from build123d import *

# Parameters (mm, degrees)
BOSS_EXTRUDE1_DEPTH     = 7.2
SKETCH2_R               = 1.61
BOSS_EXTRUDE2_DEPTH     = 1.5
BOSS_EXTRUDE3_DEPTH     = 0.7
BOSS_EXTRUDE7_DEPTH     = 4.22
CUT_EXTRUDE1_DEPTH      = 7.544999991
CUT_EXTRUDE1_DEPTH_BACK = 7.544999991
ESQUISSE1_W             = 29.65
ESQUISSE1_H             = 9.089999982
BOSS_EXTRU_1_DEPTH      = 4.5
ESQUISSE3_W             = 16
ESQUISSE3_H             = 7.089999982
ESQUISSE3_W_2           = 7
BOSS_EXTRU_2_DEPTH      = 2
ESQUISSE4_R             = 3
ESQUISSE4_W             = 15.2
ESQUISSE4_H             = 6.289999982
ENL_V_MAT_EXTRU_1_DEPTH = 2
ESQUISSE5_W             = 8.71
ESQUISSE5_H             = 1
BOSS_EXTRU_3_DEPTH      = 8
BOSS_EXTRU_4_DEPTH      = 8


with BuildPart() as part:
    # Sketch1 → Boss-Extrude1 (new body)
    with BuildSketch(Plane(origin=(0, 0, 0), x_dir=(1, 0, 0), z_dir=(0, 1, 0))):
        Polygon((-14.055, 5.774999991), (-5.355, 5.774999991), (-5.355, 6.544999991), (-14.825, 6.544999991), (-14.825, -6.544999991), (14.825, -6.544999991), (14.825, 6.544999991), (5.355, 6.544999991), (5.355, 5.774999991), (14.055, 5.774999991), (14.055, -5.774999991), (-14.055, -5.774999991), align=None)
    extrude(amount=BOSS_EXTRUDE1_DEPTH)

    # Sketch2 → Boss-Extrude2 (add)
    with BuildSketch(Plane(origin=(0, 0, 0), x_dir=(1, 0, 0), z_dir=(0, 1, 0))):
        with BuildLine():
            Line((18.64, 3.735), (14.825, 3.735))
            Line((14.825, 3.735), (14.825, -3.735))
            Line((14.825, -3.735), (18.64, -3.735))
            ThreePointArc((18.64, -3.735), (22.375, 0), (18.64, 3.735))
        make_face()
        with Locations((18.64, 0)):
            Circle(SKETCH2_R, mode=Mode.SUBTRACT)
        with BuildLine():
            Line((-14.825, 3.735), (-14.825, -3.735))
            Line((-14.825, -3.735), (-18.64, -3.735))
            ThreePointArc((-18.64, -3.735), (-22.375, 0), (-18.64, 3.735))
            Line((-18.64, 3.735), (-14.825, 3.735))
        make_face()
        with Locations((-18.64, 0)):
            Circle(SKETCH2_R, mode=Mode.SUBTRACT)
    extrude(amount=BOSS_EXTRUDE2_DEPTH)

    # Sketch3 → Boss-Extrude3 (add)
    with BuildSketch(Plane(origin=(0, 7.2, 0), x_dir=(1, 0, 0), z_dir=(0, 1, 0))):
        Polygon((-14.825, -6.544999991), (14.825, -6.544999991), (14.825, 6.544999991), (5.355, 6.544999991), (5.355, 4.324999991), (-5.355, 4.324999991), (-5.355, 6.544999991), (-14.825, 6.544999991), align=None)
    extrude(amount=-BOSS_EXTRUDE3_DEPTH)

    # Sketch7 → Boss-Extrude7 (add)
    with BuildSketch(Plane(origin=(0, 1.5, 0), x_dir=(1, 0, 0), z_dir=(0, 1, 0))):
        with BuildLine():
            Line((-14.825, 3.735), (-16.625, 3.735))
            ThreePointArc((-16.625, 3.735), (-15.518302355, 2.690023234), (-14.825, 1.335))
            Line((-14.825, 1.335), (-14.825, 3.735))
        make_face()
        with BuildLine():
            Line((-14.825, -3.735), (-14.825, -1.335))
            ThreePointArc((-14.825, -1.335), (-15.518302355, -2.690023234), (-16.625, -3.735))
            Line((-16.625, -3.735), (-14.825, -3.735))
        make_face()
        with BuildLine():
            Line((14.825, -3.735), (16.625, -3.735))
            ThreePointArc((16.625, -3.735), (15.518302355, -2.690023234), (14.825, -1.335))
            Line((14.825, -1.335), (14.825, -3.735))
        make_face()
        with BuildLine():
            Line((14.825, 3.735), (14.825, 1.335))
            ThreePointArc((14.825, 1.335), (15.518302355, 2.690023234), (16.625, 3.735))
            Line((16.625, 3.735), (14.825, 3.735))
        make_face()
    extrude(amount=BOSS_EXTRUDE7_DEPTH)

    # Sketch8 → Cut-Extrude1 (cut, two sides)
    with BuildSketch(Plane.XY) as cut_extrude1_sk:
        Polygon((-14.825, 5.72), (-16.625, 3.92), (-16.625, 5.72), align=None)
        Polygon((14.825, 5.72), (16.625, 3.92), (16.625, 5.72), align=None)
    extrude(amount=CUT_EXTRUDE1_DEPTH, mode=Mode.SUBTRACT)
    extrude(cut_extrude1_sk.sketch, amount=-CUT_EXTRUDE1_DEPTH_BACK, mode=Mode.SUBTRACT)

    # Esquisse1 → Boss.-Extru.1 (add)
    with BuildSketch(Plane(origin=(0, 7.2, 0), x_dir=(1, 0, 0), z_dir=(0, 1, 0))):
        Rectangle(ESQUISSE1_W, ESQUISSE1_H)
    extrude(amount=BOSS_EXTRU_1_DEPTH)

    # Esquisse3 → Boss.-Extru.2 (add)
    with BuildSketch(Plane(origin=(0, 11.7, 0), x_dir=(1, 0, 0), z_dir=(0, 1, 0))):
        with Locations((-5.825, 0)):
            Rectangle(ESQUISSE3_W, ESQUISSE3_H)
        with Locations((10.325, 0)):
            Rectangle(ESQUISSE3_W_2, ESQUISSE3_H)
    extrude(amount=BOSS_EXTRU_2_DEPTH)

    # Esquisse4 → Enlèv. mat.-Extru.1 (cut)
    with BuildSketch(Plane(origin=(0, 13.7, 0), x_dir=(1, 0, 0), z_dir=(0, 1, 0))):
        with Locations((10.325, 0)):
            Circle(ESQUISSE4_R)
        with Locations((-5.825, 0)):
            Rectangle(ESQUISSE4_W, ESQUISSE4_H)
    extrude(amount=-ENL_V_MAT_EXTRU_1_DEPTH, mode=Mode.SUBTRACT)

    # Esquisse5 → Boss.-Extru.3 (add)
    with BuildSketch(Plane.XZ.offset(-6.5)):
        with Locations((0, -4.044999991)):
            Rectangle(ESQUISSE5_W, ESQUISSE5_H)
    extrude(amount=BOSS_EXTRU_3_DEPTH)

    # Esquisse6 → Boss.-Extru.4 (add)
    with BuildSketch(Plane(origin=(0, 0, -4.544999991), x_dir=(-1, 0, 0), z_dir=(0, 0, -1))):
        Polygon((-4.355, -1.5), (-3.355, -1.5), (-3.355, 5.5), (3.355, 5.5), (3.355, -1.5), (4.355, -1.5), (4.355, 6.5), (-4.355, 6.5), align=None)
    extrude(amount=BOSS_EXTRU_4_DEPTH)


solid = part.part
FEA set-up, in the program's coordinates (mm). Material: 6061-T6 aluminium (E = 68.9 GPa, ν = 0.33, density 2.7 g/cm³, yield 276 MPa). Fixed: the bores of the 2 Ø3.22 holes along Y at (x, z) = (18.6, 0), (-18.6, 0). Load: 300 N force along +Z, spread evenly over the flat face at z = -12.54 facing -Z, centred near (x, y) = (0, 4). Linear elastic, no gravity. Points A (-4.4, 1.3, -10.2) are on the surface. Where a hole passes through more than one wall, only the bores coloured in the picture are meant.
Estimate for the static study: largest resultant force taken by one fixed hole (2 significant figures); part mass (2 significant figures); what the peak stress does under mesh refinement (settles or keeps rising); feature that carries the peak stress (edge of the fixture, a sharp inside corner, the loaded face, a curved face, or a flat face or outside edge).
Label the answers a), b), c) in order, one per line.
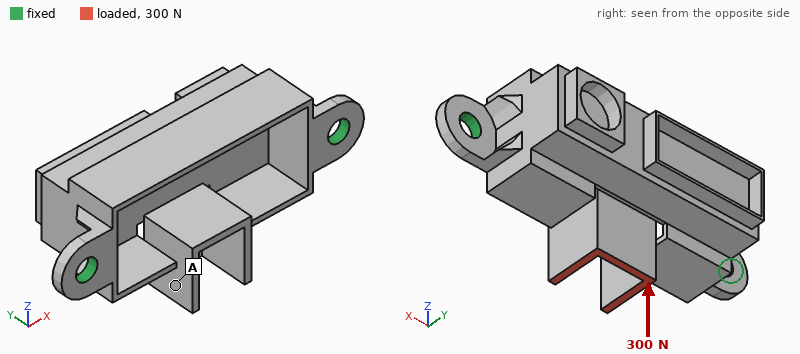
a) 150 N
b) 6.2 g
c) keeps rising
d) a sharp inside corner
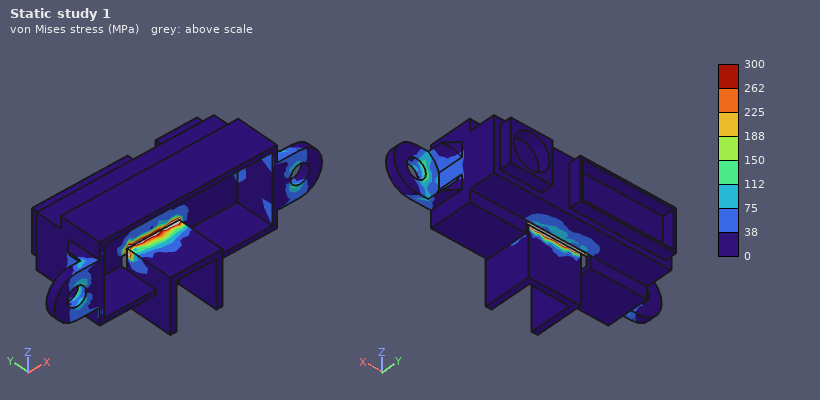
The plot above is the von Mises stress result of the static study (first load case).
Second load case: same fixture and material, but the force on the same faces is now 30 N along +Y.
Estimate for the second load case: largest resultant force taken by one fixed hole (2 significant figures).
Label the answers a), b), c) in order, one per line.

a) 17 N
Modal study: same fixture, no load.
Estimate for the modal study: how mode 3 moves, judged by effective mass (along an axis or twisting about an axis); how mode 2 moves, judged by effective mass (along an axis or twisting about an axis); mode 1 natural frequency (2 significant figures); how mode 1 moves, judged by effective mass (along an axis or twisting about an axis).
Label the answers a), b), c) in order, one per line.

a) along X
b) along Z
c) 3900 Hz
d) along Z
